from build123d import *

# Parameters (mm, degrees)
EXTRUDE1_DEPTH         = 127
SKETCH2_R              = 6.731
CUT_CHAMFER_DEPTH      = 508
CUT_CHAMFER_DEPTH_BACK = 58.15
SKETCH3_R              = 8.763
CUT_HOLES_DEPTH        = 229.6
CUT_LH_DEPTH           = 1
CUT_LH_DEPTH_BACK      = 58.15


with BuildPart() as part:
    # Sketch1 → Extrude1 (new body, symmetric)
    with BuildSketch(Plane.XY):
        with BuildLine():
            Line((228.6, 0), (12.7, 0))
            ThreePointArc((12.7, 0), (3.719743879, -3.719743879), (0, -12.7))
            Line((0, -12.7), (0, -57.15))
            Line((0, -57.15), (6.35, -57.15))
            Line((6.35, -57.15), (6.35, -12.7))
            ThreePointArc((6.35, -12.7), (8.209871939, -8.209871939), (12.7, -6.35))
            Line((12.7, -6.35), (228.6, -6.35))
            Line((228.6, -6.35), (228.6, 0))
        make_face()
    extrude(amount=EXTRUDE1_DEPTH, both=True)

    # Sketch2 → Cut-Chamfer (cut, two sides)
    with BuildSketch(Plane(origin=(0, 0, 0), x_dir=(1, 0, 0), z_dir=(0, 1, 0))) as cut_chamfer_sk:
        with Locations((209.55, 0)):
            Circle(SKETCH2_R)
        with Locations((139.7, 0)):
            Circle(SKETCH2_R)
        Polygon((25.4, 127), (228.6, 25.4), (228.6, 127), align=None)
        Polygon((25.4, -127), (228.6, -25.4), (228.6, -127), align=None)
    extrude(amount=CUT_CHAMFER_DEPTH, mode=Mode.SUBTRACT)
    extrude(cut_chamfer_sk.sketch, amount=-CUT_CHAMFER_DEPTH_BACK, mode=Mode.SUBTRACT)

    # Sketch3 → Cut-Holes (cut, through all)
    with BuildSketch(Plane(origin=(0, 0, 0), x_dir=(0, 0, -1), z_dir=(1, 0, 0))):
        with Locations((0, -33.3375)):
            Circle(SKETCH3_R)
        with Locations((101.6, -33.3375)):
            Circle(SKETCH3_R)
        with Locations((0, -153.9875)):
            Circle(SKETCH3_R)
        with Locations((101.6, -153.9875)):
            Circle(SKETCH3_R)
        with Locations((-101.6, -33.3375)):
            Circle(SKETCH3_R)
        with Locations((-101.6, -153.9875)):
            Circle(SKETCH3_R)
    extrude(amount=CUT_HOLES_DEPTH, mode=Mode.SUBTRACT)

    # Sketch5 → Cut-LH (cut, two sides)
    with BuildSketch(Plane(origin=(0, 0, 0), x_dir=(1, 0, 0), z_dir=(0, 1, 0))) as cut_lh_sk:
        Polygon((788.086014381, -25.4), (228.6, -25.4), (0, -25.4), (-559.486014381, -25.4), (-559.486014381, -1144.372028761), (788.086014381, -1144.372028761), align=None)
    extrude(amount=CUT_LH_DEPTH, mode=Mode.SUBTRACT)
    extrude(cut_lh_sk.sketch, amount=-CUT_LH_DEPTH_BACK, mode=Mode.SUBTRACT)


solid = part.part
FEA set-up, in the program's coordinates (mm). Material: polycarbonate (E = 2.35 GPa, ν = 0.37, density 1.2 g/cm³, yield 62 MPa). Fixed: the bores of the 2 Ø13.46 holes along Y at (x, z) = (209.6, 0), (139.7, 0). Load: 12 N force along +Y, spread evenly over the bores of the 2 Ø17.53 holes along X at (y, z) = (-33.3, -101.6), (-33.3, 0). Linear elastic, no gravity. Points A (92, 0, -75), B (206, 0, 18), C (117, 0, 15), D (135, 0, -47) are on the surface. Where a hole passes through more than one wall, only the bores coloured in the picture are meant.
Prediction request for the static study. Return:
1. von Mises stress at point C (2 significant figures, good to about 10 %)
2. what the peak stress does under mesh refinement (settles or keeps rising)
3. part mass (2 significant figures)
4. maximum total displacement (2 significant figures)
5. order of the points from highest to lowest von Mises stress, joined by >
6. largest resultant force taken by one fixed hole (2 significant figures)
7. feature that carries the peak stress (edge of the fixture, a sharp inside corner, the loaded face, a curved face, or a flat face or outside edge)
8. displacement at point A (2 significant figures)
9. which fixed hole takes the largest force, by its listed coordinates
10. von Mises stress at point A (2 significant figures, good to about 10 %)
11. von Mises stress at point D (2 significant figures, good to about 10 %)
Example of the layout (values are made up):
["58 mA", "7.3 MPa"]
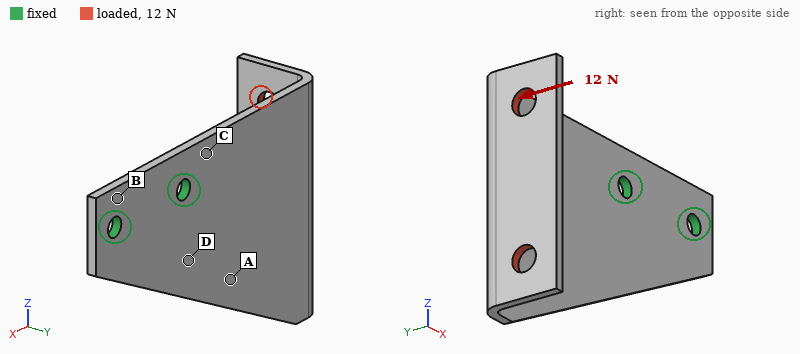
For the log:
["2.4 MPa", "keeps rising", "240 g", "3.1 mm", "C > D > A > B", "20 N", "edge of the fixture", "0.70 mm", "(139.7, 0)", "1.1 MPa", "1.7 MPa"]
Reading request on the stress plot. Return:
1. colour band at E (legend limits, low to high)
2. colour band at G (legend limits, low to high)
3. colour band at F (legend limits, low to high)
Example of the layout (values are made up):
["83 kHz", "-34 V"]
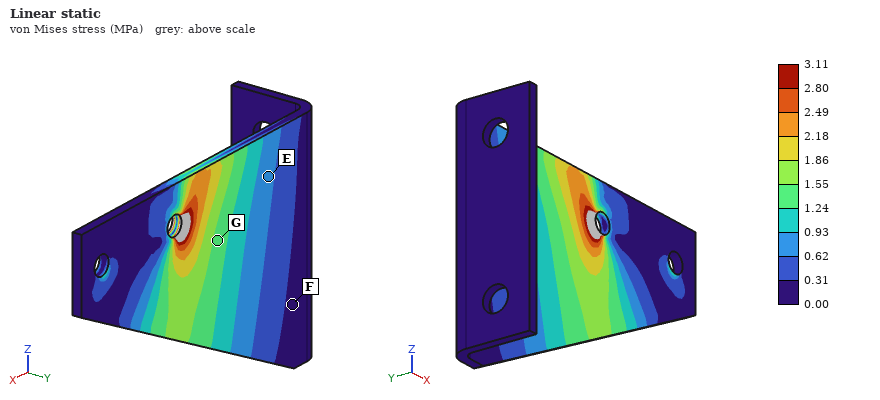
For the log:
["0.62 to 0.93 MPa", "1.24 to 1.55 MPa", "0.00 to 0.31 MPa"]
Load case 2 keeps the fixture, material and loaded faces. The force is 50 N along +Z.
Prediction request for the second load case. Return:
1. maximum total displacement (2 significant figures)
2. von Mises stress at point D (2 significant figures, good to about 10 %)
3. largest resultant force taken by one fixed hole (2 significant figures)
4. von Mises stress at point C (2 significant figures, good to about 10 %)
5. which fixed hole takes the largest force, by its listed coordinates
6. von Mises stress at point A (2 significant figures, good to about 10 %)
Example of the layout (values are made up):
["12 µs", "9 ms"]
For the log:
["3.1 mm", "1.5 MPa", "140 N", "1.9 MPa", "(139.7, 0)", "1.2 MPa"]
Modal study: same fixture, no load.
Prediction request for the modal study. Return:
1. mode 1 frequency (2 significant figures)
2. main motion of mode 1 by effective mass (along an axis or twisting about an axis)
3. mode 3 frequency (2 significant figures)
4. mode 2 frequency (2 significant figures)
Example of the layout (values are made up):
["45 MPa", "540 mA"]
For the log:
["36 Hz", "along Y", "200 Hz", "81 Hz"]
